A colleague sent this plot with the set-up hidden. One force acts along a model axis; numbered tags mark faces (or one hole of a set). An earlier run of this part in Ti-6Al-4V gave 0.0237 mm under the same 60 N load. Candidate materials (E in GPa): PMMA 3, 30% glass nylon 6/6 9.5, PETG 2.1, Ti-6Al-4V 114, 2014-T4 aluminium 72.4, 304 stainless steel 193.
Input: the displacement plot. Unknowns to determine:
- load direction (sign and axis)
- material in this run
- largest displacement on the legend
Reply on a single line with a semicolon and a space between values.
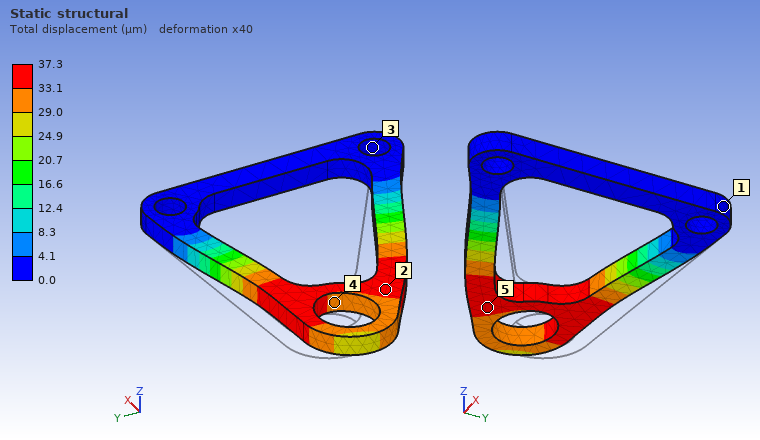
-Y; 2014-T4 aluminium; 37.3 µm
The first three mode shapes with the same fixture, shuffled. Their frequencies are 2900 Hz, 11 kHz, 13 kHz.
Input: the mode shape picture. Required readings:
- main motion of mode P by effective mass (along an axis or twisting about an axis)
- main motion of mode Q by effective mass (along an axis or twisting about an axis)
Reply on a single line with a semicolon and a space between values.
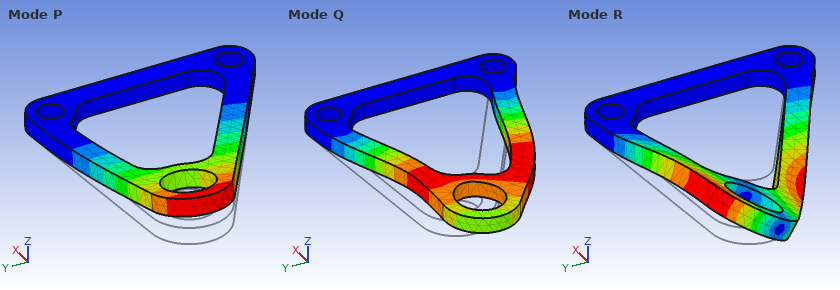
along Z; along Y
